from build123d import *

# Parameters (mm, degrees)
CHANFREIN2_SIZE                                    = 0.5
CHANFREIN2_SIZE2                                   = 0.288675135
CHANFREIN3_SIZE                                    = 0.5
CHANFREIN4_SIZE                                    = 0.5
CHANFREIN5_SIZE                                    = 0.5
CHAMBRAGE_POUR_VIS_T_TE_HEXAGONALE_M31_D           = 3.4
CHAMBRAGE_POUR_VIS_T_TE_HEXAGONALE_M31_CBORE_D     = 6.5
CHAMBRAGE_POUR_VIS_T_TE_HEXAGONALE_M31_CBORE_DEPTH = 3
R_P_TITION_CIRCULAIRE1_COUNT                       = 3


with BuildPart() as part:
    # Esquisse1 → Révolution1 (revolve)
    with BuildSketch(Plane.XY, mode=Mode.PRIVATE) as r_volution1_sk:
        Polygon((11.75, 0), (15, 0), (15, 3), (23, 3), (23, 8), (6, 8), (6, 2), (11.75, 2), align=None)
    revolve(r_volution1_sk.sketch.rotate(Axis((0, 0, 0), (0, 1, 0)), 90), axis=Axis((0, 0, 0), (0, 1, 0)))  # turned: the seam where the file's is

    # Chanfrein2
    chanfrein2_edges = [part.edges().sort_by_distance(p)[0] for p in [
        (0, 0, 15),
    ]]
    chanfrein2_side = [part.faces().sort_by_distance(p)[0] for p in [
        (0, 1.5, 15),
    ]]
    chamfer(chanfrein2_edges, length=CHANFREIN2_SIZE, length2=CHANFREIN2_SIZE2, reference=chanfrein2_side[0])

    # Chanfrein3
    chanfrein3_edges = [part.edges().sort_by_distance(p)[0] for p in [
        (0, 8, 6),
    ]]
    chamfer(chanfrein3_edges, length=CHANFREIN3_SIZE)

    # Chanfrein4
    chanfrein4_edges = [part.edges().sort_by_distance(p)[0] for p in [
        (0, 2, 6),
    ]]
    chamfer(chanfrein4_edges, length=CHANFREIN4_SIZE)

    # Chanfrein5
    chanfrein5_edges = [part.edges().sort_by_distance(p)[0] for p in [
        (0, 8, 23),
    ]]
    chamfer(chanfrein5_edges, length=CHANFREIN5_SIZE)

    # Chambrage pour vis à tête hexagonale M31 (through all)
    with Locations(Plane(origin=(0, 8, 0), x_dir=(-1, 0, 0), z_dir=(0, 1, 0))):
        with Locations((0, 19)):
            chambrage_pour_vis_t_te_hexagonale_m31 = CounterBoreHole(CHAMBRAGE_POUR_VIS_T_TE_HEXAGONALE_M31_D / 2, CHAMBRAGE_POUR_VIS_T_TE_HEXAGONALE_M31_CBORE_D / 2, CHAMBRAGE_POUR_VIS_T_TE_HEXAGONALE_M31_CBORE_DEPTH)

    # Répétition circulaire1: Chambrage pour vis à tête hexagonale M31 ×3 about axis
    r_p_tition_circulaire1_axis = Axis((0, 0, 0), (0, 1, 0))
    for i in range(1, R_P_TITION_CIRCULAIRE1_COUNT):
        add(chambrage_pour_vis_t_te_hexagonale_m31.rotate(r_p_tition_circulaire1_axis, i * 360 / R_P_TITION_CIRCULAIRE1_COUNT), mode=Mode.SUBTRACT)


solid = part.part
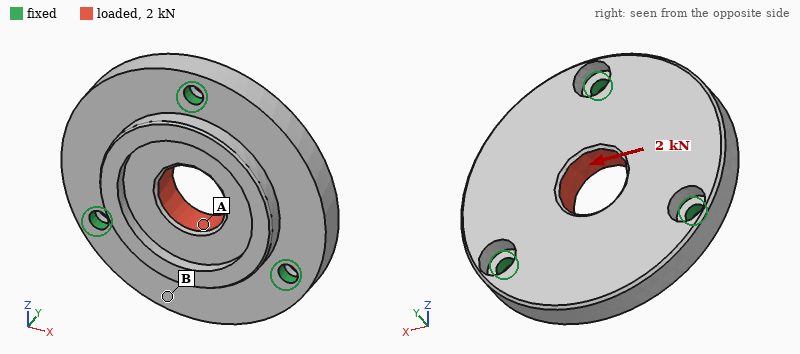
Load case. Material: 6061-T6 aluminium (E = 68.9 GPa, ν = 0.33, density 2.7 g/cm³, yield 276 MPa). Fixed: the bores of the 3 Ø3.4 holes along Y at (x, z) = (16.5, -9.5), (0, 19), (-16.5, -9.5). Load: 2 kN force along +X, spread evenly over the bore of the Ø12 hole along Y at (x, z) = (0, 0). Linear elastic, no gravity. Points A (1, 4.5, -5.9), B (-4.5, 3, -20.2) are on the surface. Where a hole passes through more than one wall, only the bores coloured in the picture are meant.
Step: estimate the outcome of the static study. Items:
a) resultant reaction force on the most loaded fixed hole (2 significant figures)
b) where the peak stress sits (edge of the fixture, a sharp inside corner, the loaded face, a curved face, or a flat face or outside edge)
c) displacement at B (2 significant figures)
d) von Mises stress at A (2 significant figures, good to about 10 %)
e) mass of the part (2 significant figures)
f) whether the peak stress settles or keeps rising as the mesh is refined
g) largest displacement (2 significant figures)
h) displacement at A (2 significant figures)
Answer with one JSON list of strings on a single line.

["680 N", "edge of the fixture", "2.0 µm", "18 MPa", "23 g", "keeps rising", "5.4 µm", "3.5 µm"]
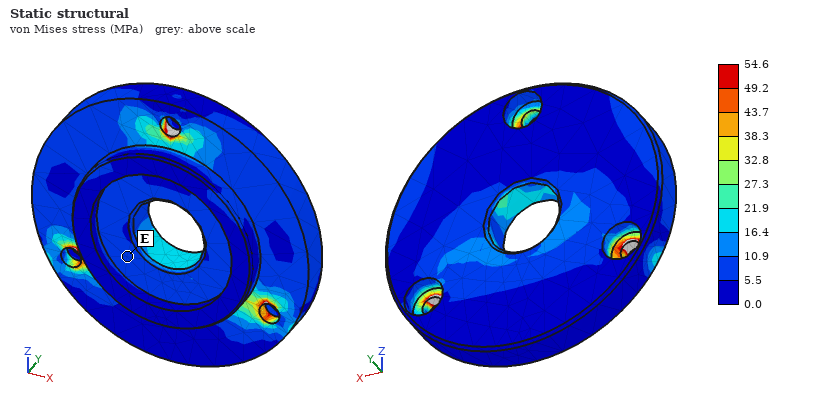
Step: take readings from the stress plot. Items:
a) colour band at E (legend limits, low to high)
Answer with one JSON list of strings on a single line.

["5.5 to 10.9 MPa"]
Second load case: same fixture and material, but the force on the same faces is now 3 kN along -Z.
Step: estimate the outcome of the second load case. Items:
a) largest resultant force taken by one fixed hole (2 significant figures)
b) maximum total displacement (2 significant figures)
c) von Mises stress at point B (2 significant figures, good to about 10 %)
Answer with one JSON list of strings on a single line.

["1.0 kN", "9.2 µm", "11 MPa"]
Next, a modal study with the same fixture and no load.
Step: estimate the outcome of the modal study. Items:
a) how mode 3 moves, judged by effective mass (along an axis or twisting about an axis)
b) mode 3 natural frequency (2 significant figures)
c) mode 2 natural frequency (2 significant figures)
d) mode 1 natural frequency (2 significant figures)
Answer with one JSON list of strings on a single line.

["along Y", "14 kHz", "11 kHz", "11 kHz"]
